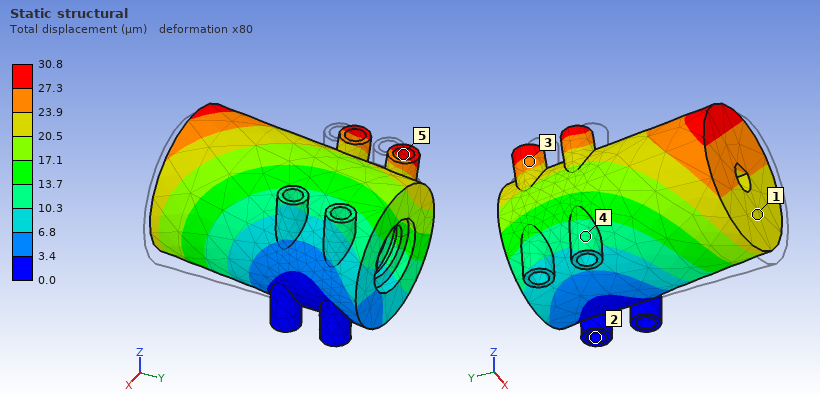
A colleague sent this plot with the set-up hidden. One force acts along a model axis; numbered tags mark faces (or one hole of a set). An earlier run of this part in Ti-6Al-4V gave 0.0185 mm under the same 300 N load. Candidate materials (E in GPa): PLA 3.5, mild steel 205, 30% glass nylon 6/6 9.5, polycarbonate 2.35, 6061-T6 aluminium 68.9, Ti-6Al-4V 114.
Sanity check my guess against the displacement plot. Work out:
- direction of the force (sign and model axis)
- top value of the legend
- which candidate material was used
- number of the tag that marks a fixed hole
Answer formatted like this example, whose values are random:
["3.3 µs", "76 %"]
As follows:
["+Y", "30.8 µm", "6061-T6 aluminium", "2"]
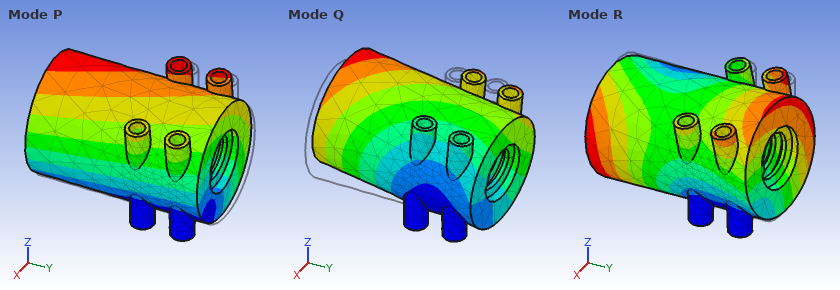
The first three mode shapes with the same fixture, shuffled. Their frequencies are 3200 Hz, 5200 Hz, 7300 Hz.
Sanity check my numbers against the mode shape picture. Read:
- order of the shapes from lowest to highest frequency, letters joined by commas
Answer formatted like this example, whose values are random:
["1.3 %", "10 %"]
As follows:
["P, Q, R"]
